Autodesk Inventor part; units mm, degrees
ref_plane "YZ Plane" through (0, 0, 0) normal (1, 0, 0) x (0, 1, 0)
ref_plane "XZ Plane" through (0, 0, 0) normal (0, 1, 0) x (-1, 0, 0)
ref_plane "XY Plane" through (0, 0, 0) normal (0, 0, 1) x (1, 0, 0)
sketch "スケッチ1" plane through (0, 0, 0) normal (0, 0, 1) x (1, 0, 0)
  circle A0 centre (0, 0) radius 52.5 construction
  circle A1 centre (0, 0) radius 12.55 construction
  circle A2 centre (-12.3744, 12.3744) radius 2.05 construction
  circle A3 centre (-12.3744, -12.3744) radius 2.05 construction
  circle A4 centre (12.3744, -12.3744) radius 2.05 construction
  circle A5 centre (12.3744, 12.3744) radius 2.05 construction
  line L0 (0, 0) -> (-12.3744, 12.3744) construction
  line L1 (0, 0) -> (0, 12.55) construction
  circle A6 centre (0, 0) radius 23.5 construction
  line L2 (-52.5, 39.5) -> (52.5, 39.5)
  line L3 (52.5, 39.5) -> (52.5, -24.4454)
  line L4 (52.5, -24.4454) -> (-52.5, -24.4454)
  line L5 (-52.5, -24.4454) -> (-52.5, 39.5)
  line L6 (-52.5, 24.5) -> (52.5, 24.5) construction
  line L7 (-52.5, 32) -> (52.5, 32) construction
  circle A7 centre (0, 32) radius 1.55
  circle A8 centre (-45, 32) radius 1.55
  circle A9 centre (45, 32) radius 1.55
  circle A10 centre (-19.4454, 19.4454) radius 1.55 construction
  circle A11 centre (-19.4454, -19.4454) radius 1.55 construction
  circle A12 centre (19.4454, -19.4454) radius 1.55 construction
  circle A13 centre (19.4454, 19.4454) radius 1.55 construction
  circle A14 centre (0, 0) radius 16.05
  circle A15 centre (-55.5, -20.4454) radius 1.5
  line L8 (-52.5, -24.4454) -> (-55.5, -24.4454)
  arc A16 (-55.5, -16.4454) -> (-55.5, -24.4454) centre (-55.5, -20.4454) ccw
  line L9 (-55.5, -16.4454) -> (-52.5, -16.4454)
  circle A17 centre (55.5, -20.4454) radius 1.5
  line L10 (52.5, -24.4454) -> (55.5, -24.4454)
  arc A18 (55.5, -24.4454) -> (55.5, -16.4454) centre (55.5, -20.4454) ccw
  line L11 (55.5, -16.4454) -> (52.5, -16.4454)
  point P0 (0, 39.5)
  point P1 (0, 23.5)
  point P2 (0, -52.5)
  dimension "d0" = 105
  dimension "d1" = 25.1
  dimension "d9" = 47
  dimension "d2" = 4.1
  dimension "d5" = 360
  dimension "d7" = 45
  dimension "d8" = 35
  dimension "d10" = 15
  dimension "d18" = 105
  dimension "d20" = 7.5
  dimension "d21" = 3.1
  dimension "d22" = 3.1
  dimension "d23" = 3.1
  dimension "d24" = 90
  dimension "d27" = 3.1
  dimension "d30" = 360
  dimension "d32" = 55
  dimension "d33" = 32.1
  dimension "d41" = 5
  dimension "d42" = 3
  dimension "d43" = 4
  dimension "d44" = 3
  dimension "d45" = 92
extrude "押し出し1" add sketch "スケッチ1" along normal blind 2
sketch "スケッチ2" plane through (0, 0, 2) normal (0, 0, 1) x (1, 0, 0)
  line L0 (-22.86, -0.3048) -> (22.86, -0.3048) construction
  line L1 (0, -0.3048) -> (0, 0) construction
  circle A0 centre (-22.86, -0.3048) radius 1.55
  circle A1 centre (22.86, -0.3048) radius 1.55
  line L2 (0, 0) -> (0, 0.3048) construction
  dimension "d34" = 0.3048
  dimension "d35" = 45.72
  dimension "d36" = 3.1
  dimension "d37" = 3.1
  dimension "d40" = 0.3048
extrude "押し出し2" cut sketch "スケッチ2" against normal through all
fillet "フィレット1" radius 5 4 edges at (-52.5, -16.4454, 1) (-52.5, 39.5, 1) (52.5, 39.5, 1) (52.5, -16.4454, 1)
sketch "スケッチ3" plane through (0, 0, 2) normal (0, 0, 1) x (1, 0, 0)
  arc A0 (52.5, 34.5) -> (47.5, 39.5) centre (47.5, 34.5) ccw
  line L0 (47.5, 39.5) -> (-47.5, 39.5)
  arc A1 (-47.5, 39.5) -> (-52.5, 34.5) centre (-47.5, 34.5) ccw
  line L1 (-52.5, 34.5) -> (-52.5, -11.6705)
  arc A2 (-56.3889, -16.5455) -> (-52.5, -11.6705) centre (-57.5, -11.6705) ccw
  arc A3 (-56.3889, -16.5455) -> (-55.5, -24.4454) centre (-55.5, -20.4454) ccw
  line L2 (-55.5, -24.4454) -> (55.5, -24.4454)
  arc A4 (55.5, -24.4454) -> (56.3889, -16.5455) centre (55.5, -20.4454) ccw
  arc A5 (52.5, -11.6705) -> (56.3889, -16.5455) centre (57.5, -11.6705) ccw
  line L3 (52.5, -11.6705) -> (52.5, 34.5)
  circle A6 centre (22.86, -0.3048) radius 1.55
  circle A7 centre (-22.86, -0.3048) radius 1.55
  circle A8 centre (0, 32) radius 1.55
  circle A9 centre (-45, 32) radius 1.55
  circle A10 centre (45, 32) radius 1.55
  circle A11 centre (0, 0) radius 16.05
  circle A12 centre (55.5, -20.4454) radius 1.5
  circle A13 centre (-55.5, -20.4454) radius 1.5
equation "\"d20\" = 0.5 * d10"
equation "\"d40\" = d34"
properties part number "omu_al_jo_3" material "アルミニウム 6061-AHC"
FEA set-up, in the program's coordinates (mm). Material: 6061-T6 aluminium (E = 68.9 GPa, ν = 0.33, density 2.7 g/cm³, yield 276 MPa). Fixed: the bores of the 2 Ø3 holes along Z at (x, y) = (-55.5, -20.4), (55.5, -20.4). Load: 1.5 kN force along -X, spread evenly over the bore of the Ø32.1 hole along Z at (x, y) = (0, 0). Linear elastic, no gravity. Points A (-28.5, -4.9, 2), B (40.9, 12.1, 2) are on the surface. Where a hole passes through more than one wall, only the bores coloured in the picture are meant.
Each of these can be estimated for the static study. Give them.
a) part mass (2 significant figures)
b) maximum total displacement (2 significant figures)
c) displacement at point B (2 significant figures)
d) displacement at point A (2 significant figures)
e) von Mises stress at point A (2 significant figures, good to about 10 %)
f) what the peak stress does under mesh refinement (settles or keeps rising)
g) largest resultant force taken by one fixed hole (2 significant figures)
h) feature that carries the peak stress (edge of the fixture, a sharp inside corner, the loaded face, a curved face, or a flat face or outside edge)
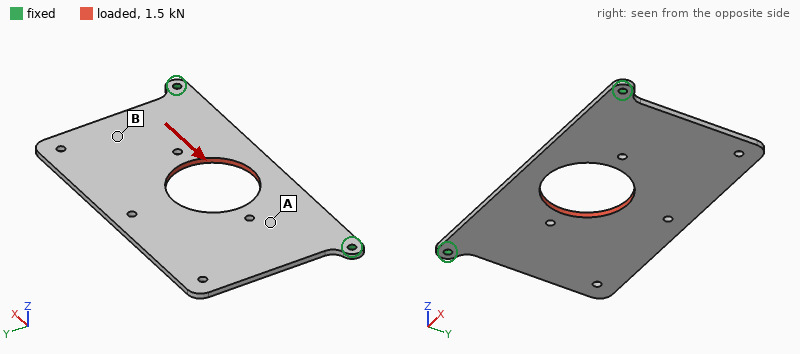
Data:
32 g
26 µm
21 µm
16 µm
13 MPa
keeps rising
800 N
edge of the fixture
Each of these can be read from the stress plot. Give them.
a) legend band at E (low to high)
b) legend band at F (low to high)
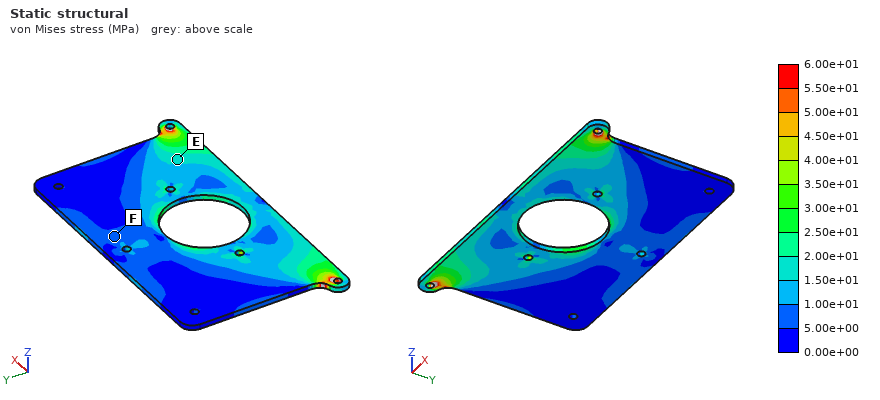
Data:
1.50e+01 to 2.00e+01 MPa
5.00e+00 to 1.00e+01 MPa
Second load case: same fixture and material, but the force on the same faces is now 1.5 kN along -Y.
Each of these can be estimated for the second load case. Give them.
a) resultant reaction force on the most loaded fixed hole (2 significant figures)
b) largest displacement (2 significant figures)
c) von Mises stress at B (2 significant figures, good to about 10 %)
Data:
890 N
47 µm
15 MPa
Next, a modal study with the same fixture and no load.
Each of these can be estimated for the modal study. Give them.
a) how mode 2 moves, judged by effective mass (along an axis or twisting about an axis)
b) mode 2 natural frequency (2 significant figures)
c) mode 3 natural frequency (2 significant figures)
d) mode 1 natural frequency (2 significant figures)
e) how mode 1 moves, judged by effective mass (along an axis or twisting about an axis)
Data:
twisting about Y
640 Hz
840 Hz
230 Hz
along Z
